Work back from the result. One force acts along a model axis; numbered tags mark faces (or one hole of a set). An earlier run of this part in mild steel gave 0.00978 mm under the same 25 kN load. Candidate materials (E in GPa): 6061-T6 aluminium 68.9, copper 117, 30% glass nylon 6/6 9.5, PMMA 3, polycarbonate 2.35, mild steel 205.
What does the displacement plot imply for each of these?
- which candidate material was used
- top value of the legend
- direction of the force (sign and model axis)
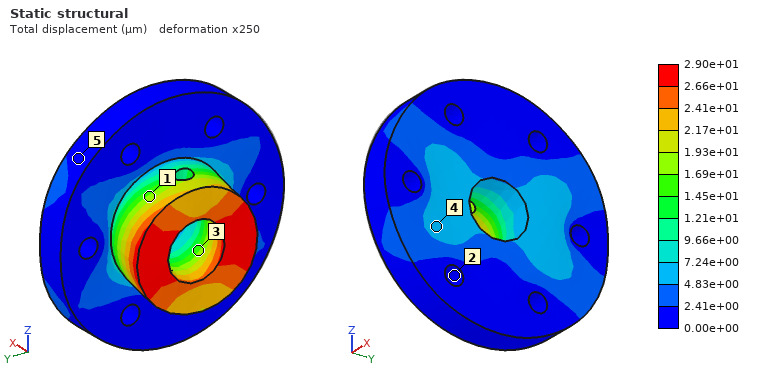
6061-T6 aluminium
2.90e+01 µm
+Y
